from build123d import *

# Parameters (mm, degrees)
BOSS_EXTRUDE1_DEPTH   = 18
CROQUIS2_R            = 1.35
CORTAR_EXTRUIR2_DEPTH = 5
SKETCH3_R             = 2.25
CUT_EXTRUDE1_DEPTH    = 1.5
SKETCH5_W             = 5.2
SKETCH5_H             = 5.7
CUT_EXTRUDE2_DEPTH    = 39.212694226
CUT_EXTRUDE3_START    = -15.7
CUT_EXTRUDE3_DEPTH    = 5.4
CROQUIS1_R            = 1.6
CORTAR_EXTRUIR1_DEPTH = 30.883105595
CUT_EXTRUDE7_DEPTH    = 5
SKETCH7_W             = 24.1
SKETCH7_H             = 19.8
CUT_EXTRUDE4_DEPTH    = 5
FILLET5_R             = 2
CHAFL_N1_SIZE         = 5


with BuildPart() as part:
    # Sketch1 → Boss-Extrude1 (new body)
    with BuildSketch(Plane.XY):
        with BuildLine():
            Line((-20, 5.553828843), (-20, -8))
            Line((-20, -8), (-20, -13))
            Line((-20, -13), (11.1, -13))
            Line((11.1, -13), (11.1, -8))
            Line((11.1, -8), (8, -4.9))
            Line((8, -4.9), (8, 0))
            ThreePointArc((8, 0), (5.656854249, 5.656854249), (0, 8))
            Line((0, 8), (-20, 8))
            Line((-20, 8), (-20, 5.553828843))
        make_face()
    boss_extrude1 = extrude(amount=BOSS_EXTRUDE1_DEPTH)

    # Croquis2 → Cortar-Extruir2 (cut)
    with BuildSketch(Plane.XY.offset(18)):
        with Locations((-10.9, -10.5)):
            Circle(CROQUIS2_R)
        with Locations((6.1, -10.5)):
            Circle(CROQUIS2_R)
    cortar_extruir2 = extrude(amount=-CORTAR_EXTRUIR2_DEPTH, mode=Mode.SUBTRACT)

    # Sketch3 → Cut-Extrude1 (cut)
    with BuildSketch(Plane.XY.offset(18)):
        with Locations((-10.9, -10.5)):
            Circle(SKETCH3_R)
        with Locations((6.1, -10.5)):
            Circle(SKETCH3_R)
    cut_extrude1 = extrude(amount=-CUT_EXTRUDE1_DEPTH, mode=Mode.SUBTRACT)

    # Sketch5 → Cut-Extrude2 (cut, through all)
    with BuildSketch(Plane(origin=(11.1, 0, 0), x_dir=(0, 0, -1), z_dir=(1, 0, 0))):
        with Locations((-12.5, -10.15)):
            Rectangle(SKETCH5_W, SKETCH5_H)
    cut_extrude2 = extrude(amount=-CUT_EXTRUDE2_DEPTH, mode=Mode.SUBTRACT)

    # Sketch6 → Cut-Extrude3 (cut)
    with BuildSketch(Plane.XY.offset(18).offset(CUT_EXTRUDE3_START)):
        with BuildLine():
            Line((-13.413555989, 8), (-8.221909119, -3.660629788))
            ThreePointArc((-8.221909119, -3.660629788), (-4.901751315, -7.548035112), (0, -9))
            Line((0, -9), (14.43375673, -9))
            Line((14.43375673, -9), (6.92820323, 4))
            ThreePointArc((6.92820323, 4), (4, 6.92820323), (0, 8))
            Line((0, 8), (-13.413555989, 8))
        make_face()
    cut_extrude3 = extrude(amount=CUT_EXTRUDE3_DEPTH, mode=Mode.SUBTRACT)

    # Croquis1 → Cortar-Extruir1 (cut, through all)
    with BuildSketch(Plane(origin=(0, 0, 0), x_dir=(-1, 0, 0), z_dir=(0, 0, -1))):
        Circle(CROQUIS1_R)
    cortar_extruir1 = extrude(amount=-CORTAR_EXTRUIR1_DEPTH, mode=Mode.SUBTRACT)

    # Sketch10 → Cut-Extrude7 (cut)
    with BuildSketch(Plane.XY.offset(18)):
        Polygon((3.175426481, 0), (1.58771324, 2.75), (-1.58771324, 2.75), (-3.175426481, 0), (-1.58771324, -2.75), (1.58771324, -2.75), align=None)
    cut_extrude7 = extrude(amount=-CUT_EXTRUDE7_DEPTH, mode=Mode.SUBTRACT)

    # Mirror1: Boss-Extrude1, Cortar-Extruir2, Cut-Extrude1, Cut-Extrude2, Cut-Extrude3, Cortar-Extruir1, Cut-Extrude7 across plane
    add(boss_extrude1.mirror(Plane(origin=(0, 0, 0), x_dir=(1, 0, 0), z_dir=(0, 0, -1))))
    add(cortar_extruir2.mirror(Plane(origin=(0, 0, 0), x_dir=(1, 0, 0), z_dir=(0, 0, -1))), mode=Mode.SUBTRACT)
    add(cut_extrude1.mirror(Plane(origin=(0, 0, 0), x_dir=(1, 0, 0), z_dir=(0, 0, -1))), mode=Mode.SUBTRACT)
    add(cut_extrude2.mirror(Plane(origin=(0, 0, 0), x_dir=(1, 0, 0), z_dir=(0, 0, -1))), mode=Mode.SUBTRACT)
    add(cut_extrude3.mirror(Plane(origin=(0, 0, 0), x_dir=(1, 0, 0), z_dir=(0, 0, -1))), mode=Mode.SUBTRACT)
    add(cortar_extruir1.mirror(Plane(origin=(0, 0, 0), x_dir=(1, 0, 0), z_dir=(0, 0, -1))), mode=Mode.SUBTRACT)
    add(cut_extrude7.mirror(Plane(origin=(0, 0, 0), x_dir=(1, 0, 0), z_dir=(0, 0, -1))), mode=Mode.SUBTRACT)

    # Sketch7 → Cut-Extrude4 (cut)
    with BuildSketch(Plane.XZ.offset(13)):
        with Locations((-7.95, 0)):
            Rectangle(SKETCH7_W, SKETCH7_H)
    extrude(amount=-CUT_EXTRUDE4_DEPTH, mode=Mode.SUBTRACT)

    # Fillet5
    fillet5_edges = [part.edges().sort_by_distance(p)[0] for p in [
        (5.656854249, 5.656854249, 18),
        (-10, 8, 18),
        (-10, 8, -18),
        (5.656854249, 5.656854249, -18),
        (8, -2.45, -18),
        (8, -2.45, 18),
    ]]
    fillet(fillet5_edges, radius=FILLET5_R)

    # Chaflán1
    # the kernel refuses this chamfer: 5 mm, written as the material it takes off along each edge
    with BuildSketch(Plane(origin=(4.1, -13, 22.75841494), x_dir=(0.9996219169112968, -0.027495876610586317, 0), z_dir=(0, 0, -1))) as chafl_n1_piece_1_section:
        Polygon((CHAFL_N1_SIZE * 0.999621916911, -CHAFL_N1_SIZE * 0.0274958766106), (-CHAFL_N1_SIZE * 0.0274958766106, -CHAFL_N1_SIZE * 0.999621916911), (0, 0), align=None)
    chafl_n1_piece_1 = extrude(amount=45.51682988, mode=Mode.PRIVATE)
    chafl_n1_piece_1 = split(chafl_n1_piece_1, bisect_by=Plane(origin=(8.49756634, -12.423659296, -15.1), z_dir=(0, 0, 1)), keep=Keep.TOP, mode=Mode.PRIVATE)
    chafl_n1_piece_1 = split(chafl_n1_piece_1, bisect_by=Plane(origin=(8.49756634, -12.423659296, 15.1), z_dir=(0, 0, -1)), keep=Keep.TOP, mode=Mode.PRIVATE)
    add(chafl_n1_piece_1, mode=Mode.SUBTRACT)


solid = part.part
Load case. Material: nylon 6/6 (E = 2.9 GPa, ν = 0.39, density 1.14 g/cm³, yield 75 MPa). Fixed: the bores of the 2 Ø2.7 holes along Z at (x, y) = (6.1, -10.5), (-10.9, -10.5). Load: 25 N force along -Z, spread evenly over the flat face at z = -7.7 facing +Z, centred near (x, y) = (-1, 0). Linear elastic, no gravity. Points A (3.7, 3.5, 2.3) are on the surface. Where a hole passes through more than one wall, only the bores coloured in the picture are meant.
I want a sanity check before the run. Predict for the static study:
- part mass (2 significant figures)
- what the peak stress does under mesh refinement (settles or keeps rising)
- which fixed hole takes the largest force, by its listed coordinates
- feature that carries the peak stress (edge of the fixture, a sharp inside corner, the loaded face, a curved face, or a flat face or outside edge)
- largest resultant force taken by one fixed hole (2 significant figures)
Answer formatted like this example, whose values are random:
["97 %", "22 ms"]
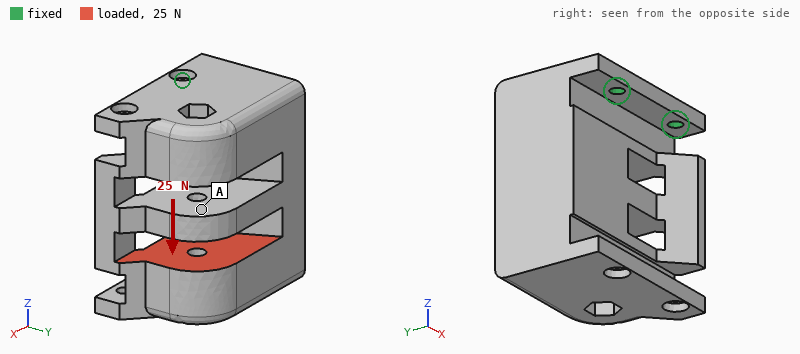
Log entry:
["15 g", "keeps rising", "(6.1, -10.5)", "edge of the fixture", "15 N"]
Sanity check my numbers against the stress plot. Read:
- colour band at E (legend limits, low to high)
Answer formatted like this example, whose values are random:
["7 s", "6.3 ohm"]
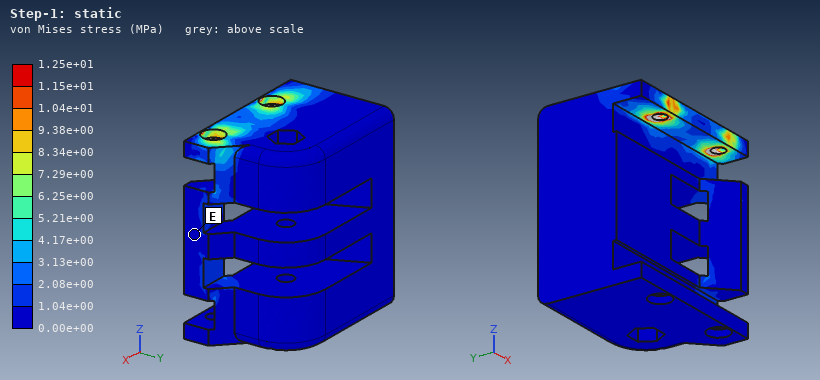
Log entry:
["0.00e+00 to 1.04e+00 MPa"]
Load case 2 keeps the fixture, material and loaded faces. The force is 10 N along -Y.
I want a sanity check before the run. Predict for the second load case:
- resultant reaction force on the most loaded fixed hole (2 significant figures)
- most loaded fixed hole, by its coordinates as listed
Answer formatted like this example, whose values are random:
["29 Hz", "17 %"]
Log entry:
["6.1 N", "(6.1, -10.5)"]
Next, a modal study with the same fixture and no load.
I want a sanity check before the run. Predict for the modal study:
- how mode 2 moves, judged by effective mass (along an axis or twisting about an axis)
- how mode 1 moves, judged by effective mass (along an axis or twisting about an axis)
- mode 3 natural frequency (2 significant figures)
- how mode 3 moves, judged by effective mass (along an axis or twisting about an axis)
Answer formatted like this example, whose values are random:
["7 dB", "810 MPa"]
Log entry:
["along X", "along Y", "2100 Hz", "along Z"]
